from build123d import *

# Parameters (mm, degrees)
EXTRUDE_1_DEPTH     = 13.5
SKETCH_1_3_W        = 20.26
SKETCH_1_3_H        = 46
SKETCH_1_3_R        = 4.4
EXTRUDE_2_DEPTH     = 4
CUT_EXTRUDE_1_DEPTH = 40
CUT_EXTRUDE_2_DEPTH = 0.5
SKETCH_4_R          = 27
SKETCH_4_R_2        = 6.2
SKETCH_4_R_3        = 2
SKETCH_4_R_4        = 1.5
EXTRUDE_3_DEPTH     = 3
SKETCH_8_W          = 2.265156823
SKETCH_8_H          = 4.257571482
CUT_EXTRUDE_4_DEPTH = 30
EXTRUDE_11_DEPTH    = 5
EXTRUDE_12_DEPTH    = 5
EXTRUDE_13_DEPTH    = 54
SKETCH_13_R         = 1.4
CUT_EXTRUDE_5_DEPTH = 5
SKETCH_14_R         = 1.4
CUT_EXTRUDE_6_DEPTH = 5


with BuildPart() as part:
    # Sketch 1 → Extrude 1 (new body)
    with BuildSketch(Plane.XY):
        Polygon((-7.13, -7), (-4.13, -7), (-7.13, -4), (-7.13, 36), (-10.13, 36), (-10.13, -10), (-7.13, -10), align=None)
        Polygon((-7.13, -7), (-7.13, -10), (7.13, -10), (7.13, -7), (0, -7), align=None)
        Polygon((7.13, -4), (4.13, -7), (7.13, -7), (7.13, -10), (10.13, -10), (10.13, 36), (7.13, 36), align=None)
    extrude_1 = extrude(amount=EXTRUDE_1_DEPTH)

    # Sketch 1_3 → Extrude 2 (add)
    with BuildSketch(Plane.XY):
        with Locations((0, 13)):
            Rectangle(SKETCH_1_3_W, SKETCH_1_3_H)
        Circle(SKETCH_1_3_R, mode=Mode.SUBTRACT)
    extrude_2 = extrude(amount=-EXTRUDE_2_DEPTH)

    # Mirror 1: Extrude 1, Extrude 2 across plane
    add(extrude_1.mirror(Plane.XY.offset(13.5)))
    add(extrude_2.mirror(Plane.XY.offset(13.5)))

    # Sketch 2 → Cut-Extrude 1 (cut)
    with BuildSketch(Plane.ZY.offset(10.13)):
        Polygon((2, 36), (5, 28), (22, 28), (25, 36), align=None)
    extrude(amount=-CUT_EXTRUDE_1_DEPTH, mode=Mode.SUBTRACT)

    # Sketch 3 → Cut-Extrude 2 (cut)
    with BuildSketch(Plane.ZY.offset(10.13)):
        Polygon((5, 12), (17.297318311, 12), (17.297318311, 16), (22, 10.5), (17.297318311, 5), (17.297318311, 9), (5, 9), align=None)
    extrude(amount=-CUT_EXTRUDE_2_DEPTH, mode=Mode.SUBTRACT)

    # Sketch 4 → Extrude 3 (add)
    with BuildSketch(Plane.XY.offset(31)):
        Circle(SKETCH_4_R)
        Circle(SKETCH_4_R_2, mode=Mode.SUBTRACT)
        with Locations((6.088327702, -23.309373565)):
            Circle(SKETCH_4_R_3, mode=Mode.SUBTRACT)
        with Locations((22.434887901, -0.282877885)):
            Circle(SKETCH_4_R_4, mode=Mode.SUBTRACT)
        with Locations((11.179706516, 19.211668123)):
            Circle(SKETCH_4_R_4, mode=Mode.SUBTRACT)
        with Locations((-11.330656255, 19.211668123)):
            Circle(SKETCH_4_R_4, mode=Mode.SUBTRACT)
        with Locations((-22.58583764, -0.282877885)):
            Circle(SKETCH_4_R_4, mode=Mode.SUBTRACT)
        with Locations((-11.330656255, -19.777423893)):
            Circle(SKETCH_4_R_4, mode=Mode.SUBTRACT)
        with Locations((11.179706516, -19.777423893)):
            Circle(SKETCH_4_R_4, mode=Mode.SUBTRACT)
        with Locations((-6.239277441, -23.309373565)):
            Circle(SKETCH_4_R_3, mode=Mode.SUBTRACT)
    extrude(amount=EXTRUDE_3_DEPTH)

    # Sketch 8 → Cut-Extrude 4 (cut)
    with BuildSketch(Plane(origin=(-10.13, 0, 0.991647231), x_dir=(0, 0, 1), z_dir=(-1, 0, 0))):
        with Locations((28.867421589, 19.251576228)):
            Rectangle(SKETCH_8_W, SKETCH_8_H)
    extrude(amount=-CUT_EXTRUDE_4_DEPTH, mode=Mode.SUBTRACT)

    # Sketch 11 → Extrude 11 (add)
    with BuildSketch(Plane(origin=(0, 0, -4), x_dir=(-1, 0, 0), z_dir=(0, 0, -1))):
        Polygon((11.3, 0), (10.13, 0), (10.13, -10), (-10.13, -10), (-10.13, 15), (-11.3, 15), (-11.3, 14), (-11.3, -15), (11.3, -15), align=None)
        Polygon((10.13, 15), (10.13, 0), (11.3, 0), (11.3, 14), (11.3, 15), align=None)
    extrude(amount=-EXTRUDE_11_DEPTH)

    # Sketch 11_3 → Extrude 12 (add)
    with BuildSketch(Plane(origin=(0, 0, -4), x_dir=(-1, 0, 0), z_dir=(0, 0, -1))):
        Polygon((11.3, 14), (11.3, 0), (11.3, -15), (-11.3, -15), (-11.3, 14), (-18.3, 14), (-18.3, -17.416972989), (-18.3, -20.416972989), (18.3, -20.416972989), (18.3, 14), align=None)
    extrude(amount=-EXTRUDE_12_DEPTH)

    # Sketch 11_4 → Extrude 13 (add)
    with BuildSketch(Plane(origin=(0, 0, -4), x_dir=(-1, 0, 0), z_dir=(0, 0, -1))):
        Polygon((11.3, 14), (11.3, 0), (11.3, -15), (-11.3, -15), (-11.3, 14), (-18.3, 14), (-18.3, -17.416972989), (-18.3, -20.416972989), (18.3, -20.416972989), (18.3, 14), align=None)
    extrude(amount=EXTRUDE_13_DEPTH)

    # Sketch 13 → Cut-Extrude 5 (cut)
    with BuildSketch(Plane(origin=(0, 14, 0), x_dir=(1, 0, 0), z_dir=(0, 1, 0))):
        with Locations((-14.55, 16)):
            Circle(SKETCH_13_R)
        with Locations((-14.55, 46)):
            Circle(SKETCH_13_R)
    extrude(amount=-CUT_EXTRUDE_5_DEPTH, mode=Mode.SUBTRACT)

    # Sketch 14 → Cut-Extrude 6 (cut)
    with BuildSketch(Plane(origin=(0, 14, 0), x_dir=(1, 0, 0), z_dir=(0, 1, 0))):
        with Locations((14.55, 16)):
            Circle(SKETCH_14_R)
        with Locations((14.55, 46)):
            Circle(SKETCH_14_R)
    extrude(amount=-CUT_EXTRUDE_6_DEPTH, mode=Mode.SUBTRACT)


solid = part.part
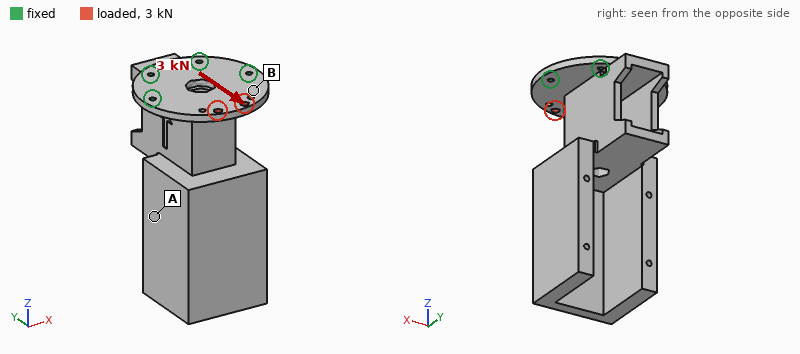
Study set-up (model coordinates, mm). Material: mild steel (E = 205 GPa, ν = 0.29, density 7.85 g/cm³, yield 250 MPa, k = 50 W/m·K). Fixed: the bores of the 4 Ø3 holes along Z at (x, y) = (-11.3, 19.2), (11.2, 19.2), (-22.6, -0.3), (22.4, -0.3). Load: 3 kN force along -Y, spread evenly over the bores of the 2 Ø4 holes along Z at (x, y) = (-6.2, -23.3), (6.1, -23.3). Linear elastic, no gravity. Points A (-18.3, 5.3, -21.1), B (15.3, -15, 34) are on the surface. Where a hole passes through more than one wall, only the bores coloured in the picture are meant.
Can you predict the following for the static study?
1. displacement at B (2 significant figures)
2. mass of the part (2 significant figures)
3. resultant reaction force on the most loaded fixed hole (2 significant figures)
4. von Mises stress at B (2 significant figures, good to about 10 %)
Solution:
2.8 µm
450 g
890 N
21 MPa
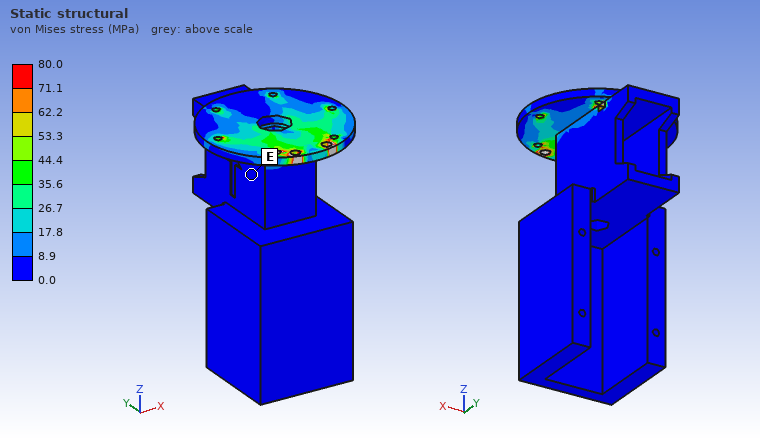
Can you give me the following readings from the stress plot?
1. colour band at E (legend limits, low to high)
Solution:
0.0 to 8.9 MPa
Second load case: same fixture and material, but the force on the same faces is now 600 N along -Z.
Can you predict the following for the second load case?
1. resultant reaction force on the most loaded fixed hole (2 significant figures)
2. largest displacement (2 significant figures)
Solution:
550 N
0.10 mm
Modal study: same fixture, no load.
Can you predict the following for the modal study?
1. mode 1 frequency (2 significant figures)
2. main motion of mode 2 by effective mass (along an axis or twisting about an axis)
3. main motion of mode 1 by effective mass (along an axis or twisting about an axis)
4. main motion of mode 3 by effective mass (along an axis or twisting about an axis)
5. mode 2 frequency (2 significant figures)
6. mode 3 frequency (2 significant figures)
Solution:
730 Hz
along X
along Y
twisting about Z
810 Hz
2600 Hz
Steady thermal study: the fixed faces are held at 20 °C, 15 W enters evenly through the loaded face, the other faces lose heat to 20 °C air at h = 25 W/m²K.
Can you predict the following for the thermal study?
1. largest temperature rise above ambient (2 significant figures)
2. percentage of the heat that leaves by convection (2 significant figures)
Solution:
76 K
30 %
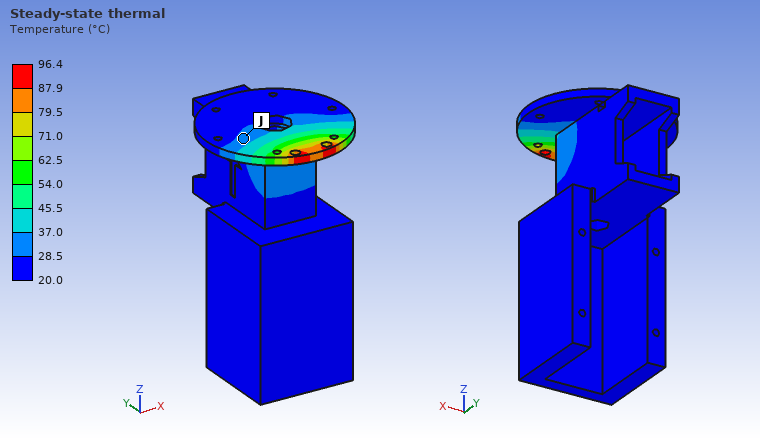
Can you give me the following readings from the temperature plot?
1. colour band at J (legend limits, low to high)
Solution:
28.5 to 37.0 °C
